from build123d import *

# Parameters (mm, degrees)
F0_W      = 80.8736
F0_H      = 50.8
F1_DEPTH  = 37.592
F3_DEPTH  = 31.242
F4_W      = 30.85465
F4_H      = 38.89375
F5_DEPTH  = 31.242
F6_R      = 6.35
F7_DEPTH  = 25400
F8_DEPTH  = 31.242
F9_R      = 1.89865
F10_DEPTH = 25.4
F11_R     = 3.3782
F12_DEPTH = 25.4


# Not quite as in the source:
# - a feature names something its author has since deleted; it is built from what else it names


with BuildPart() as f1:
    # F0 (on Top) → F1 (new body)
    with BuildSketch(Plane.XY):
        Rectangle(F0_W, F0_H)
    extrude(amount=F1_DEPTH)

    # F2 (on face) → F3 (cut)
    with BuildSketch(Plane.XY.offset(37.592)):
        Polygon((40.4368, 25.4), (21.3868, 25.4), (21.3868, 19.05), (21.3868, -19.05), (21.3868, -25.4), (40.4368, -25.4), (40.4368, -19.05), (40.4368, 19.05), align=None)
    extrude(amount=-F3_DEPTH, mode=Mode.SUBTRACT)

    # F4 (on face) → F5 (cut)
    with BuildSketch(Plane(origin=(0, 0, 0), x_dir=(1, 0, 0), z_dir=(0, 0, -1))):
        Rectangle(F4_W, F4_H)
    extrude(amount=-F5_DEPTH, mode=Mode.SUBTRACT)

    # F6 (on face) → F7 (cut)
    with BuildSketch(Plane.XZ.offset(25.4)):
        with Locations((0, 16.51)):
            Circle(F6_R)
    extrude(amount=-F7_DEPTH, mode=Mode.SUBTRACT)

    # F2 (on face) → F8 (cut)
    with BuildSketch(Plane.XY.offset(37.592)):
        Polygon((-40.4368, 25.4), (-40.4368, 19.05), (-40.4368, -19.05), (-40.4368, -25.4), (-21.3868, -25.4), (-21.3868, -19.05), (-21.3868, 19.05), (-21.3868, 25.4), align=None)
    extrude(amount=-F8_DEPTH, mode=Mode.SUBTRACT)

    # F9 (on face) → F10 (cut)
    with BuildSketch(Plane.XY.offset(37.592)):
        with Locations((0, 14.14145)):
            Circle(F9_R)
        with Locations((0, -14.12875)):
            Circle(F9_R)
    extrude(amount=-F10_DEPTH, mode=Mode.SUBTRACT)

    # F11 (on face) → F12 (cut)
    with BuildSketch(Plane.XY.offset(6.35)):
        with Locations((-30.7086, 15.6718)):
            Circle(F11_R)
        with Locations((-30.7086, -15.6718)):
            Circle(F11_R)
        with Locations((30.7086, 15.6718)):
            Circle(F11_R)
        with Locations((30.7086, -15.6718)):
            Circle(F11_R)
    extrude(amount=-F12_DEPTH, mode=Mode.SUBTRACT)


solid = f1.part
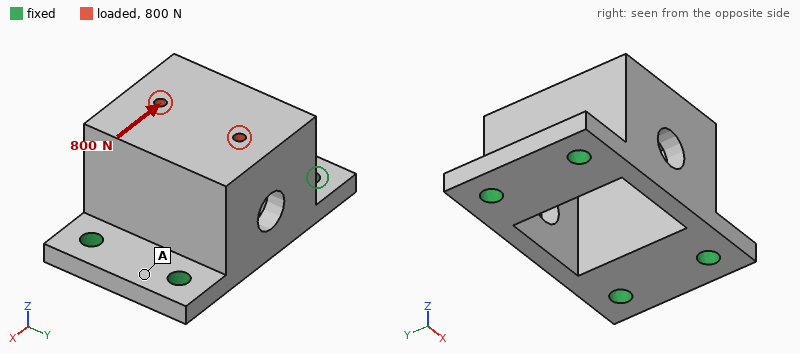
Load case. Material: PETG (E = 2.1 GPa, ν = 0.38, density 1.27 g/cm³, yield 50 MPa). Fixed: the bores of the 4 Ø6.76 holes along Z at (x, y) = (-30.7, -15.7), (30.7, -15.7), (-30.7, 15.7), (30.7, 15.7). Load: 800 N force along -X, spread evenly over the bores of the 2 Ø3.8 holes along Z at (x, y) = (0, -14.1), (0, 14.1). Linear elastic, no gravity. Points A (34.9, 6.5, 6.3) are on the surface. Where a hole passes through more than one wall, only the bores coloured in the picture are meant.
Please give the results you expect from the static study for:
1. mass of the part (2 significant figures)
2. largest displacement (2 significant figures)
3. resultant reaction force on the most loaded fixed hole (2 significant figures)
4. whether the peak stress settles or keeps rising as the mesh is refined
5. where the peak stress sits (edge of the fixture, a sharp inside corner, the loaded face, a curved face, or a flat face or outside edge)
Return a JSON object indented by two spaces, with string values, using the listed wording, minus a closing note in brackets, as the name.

{
  "mass of the part": "68 g",
  "largest displacement": "0.21 mm",
  "resultant reaction force on the most loaded fixed hole": "320 N",
  "whether the peak stress settles or keeps rising as the mesh is refined": "keeps rising",
  "where the peak stress sits": "edge of the fixture"
}
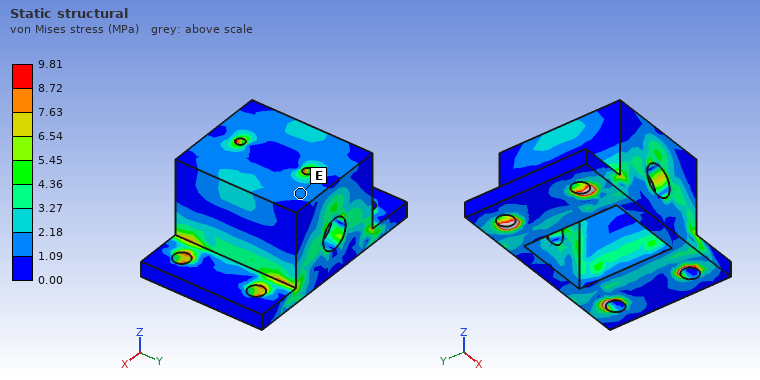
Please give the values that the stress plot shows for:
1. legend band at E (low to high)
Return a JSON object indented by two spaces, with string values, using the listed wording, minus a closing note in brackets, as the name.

{
  "legend band at E": "1.09 to 2.18 MPa"
}
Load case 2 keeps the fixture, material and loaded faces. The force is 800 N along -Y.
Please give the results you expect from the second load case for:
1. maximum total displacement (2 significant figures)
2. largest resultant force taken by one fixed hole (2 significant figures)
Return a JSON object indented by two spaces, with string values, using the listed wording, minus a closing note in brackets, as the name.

{
  "maximum total displacement": "0.37 mm",
  "largest resultant force taken by one fixed hole": "440 N"
}
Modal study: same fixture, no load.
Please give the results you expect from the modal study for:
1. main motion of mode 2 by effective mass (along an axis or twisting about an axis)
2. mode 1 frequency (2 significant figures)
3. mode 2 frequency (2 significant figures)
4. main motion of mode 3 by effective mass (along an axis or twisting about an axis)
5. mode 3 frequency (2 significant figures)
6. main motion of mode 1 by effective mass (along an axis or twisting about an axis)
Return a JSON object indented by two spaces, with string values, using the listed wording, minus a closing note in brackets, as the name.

{
  "main motion of mode 2 by effective mass": "along X",
  "mode 1 frequency": "1400 Hz",
  "mode 2 frequency": "2000 Hz",
  "main motion of mode 3 by effective mass": "along Z",
  "mode 3 frequency": "2400 Hz",
  "main motion of mode 1 by effective mass": "along Y"
}
